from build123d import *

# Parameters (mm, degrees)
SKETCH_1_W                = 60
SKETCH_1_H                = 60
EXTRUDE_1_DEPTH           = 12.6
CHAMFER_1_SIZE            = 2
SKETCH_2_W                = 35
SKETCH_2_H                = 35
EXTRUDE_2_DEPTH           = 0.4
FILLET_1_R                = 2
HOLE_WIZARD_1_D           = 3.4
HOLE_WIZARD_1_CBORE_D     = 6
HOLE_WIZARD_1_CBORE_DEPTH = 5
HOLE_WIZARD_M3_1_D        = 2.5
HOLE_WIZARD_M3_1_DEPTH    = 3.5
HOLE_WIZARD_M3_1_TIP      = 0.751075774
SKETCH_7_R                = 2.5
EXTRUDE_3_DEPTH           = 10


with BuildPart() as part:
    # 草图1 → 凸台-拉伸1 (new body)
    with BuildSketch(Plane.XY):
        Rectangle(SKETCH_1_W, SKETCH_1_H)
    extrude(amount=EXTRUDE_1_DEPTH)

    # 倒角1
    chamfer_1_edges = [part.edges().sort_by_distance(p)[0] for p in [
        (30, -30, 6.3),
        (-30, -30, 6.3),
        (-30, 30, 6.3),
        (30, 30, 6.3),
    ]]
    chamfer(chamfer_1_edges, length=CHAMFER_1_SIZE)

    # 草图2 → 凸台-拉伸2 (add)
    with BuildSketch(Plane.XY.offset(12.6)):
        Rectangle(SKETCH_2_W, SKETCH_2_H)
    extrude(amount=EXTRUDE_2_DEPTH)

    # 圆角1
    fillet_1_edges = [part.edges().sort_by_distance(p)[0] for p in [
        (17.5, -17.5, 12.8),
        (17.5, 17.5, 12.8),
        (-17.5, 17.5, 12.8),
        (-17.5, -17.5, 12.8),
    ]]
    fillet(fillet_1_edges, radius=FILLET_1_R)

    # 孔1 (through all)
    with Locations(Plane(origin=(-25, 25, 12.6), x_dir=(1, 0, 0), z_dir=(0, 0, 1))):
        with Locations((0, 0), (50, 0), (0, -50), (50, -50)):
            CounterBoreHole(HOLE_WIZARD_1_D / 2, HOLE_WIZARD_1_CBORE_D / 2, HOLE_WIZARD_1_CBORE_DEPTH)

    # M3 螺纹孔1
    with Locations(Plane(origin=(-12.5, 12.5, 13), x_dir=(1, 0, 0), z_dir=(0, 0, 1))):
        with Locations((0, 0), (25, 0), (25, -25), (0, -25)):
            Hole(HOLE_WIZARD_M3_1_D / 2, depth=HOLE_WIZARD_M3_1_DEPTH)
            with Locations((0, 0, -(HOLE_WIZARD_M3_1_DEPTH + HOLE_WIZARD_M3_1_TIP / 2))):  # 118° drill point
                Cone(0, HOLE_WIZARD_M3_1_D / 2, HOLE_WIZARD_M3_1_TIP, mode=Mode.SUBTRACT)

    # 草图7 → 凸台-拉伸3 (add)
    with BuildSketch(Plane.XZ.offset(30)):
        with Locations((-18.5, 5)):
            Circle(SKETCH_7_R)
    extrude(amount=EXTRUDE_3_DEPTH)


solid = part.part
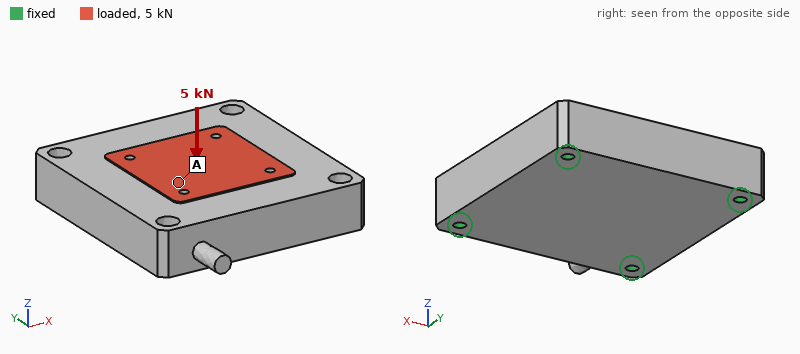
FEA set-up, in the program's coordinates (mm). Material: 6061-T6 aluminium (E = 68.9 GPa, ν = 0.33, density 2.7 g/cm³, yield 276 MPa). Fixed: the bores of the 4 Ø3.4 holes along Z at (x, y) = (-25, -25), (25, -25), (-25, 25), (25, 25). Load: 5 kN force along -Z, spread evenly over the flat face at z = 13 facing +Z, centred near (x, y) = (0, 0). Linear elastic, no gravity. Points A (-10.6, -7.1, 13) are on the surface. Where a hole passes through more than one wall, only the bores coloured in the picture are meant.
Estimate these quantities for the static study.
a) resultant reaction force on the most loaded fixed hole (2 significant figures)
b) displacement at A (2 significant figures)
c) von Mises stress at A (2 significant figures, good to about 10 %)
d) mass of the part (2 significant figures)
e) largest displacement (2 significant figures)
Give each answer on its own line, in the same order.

1.5 kN
16 µm
14 MPa
120 g
18 µm
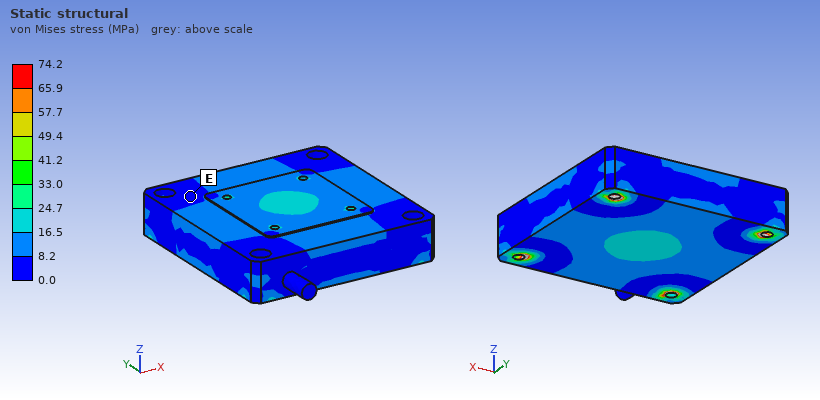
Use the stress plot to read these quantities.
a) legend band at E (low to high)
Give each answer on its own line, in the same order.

0.0 to 8.2 MPa
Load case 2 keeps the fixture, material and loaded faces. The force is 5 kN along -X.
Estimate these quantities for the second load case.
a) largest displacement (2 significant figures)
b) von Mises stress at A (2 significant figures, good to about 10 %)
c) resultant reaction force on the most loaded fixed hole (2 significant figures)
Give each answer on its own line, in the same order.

5.6 µm
8.8 MPa
1.5 kN
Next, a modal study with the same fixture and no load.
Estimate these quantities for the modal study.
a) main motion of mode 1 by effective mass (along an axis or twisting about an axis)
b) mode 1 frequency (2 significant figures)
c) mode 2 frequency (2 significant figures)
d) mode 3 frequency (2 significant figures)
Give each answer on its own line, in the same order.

along Z
11 kHz
17 kHz
17 kHz
